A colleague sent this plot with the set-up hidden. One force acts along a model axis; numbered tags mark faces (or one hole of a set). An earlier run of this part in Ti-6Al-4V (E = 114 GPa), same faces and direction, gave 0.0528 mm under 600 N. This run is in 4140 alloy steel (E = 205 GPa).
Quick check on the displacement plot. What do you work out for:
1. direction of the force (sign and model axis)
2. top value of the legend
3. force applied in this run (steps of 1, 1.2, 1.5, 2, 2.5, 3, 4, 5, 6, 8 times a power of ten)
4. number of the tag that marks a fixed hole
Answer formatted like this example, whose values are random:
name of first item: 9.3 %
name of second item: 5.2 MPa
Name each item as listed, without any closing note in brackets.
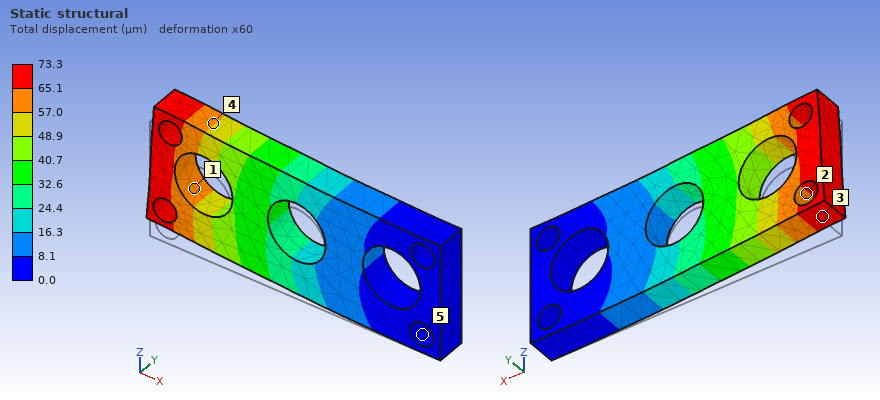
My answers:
direction of the force: +Z
top value of the legend: 73.3 µm
force applied in this run: 1.5 kN
number of the tag that marks a fixed hole: 5
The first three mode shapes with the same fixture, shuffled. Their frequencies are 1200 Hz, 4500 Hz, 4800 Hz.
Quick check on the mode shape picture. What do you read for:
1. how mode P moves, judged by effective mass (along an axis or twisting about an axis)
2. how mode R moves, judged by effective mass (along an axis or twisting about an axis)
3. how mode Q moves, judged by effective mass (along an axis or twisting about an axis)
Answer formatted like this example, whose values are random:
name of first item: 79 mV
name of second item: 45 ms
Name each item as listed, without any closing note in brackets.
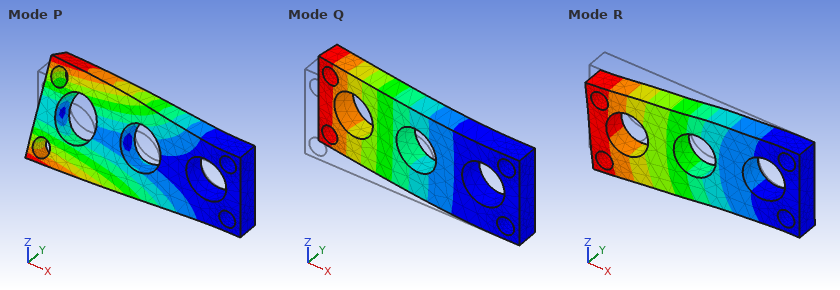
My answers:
how mode P moves, judged by effective mass: twisting about X
how mode R moves, judged by effective mass: along Z
how mode Q moves, judged by effective mass: along Y
